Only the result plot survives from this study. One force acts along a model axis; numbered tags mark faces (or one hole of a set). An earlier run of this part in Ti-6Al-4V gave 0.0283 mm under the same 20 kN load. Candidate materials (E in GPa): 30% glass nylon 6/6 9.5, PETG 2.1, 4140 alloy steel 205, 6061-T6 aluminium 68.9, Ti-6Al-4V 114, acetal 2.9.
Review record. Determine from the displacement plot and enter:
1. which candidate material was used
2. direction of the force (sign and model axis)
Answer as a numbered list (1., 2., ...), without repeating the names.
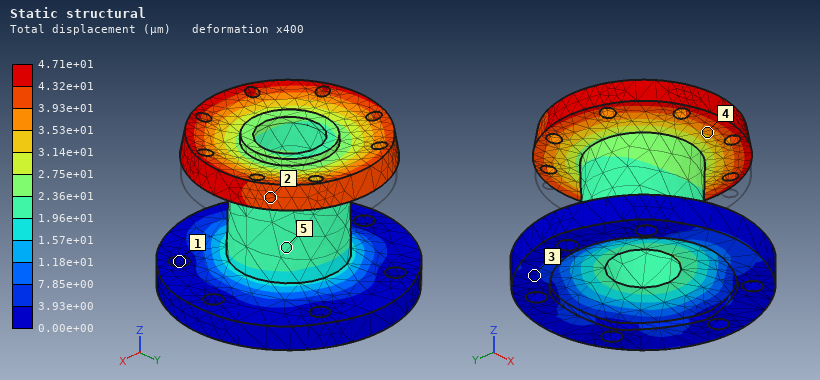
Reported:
1. 6061-T6 aluminium
2. +Z
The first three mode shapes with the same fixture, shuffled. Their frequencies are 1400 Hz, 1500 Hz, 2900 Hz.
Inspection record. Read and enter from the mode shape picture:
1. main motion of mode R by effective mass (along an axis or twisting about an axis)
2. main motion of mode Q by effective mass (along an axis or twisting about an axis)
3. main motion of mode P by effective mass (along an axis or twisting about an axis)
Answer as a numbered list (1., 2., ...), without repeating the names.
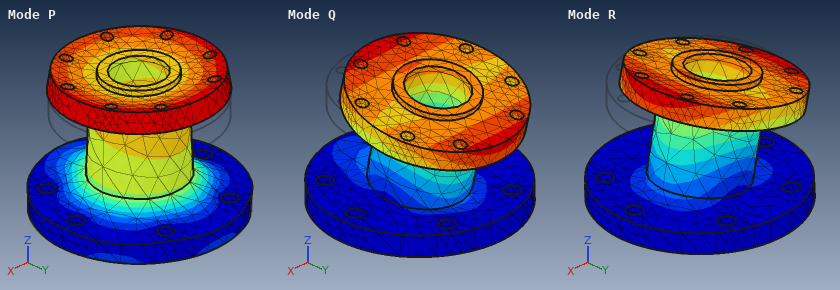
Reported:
1. along X
2. along Y
3. along Z
